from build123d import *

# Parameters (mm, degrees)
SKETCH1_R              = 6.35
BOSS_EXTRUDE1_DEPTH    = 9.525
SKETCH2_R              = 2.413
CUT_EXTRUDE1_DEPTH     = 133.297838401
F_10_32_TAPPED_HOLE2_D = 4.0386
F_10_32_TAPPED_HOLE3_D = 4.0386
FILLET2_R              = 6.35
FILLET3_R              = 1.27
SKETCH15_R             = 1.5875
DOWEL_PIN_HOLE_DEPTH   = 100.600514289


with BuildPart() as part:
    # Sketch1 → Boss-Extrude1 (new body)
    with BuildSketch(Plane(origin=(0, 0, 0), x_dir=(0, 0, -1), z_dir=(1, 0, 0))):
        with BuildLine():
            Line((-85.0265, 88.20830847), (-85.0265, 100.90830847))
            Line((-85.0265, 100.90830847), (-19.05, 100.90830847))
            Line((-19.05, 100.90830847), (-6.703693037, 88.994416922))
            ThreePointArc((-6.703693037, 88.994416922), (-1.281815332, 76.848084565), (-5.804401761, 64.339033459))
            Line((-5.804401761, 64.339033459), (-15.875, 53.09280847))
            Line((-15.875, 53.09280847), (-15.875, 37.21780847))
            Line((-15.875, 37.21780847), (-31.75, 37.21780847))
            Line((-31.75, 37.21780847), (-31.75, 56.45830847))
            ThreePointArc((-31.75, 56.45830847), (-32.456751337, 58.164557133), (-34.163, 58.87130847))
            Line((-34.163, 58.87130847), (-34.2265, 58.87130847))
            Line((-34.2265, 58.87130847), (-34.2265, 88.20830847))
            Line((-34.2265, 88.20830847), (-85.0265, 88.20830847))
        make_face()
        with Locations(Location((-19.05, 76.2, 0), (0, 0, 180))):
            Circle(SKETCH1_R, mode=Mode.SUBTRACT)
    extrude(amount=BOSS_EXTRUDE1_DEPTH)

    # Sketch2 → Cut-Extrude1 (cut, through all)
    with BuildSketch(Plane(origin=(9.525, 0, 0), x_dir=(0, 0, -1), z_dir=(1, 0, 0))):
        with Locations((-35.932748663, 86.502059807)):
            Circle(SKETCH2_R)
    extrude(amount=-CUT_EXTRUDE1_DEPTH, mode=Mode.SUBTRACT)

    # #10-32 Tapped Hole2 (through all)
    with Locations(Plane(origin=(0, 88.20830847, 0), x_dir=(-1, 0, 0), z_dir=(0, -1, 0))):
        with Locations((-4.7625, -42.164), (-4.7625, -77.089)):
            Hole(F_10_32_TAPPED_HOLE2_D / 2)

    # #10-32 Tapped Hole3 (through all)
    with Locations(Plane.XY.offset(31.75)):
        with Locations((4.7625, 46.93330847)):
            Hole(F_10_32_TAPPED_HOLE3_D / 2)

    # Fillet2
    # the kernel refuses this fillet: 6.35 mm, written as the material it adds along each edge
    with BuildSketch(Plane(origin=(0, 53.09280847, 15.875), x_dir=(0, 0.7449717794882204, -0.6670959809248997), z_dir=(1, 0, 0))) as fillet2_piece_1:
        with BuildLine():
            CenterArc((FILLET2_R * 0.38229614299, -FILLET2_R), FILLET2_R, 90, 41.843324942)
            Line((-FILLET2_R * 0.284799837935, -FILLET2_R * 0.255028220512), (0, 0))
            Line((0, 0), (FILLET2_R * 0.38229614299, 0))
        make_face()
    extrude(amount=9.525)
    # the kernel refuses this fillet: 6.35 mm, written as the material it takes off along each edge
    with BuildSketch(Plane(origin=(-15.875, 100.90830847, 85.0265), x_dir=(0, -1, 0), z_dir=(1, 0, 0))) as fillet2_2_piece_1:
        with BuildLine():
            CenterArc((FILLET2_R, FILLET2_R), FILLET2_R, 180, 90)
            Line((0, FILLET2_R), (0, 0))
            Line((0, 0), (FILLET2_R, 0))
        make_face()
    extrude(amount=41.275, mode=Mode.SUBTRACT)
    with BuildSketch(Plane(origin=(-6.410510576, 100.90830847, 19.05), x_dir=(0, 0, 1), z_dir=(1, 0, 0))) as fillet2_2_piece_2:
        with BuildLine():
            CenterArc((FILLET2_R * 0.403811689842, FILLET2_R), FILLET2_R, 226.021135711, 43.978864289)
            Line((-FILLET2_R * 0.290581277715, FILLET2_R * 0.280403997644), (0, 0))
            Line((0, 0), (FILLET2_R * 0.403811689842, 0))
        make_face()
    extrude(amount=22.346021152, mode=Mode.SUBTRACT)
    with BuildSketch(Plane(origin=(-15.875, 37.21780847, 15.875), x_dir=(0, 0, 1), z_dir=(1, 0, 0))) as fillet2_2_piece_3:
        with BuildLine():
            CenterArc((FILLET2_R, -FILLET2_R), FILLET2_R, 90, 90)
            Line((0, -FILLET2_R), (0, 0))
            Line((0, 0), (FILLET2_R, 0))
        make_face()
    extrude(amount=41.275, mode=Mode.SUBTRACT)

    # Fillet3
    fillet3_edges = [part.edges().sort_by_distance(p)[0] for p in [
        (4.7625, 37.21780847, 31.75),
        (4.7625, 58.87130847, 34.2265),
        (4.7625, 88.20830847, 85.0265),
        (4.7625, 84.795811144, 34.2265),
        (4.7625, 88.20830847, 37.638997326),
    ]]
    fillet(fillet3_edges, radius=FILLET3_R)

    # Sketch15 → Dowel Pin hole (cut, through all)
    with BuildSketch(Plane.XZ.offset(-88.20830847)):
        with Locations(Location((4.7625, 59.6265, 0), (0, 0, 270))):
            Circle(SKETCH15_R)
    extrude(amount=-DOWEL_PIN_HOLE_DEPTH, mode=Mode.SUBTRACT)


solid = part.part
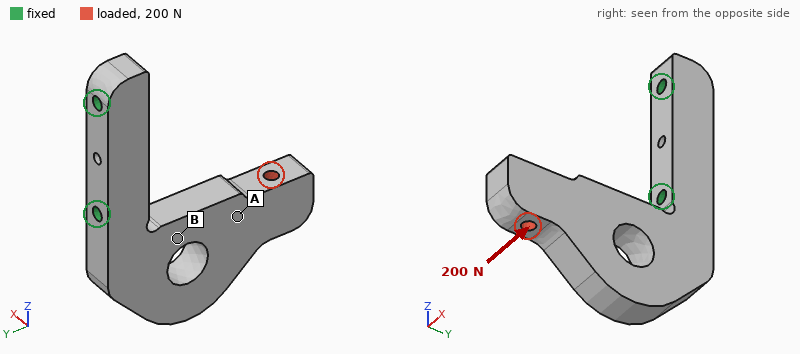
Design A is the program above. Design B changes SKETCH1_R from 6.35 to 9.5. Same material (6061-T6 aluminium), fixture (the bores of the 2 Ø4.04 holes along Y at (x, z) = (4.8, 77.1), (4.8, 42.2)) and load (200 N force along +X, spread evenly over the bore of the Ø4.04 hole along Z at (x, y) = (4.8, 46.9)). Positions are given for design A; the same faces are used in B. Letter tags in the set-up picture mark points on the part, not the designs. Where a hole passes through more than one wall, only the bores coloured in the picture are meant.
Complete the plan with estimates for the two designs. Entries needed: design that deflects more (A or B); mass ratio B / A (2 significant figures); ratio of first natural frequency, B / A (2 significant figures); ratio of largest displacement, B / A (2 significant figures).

B
0.92
0.97
1.2
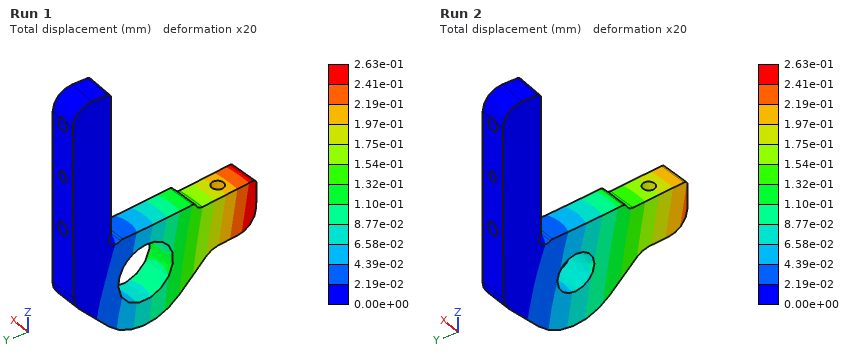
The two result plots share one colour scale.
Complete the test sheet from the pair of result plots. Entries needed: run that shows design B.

Run 1
